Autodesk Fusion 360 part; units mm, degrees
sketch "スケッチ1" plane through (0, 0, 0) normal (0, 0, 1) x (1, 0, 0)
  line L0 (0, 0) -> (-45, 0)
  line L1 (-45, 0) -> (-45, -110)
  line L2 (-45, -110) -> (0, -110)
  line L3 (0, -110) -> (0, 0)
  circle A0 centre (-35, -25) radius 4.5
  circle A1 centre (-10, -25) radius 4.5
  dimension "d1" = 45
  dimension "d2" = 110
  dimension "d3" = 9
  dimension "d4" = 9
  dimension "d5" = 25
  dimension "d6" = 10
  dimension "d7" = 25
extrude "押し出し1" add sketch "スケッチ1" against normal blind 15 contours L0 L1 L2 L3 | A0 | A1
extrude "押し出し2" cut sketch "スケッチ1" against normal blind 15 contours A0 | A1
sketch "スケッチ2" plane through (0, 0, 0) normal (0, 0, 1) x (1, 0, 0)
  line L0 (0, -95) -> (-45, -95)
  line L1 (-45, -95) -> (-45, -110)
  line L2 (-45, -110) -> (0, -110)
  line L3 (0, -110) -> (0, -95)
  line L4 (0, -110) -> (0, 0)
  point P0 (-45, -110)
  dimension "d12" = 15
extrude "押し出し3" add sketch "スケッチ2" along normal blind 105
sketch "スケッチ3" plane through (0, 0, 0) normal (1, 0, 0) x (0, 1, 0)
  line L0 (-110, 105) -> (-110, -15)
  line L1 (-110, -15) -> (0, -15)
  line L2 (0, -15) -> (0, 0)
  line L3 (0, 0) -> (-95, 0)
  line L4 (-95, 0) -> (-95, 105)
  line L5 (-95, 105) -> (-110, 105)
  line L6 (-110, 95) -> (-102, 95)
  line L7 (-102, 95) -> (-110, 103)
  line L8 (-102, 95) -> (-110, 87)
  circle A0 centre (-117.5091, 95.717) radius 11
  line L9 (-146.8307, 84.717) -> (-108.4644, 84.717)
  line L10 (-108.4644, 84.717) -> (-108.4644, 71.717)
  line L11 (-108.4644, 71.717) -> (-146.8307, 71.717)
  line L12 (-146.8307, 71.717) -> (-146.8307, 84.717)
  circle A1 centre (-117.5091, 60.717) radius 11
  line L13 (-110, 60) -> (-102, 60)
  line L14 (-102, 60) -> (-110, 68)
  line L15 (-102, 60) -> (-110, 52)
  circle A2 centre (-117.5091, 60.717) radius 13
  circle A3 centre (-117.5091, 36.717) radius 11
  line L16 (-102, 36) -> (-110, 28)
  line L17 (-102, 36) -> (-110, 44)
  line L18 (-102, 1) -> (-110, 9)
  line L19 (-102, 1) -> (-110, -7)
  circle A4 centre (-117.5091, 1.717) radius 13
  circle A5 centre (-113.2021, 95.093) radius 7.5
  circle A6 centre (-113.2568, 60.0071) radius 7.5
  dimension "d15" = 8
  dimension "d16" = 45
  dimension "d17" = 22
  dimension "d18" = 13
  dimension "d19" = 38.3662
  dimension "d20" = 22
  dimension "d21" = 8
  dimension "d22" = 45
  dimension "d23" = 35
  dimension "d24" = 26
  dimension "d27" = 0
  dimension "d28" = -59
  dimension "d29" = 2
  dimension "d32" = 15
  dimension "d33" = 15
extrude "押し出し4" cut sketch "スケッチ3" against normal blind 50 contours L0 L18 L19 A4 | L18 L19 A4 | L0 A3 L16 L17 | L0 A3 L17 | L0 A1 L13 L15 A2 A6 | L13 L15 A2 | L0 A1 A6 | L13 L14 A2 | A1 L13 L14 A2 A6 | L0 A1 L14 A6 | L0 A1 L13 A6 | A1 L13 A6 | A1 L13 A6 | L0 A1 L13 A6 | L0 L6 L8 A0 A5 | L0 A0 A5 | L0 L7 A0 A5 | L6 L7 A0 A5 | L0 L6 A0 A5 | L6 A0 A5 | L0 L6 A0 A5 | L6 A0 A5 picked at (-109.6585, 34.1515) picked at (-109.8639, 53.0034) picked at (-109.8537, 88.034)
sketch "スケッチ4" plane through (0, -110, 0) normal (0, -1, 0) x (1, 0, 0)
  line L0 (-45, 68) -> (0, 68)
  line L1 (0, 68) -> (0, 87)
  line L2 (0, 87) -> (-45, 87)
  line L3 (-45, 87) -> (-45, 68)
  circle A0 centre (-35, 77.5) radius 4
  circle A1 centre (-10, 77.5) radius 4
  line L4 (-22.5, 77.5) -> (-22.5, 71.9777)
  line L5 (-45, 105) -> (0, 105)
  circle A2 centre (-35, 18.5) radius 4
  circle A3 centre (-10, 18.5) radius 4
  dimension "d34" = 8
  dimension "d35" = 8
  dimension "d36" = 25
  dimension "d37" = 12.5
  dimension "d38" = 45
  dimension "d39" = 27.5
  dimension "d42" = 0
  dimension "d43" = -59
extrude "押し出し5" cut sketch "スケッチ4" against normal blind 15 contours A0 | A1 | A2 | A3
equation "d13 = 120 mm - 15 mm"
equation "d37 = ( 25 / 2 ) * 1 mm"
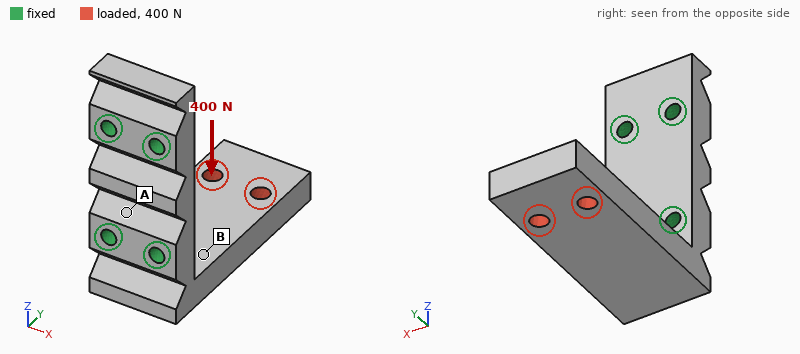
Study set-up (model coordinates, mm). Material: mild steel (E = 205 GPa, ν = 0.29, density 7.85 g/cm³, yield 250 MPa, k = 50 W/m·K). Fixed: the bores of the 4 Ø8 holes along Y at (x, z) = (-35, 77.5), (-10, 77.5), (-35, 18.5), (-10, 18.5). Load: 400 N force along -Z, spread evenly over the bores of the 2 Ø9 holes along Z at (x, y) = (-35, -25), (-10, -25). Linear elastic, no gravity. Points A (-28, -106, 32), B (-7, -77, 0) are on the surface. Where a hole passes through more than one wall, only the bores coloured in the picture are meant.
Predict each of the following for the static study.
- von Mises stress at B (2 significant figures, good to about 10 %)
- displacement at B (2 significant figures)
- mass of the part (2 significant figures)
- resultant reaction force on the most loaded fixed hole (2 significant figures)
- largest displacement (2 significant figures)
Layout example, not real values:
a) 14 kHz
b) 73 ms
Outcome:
a) 12 MPa
b) 0.020 mm
c) 1.0 kg
d) 190 N
e) 0.11 mm
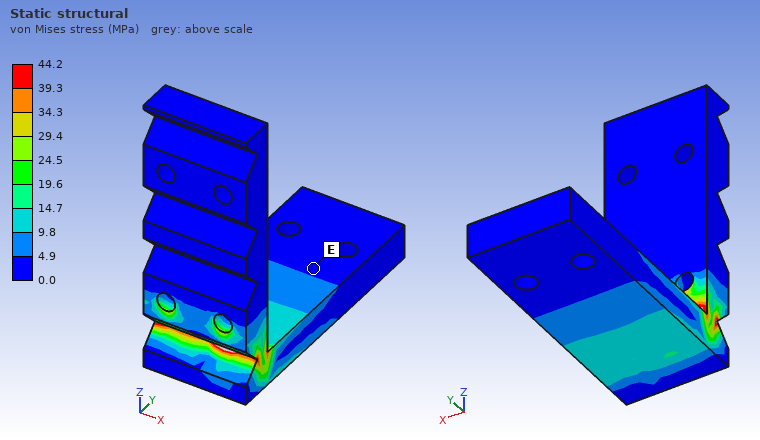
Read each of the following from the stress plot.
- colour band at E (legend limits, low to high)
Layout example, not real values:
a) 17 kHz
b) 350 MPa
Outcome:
a) 0.0 to 4.9 MPa
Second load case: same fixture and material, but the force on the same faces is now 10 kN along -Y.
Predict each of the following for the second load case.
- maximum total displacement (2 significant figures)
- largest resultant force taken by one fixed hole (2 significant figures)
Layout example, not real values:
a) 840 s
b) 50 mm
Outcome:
a) 0.31 mm
b) 5.1 kN
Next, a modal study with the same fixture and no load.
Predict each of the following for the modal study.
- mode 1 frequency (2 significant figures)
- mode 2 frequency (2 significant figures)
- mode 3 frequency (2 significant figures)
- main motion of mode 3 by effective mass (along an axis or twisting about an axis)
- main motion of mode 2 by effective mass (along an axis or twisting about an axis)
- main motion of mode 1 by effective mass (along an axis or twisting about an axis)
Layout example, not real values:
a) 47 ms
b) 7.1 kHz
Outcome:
a) 640 Hz
b) 1500 Hz
c) 4200 Hz
d) along Y
e) along X
f) along Z
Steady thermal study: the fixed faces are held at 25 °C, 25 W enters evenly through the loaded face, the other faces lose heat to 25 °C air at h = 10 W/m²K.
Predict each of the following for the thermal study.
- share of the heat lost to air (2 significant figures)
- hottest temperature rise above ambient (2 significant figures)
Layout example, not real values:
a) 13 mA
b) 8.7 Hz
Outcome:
a) 24 %
b) 65 K
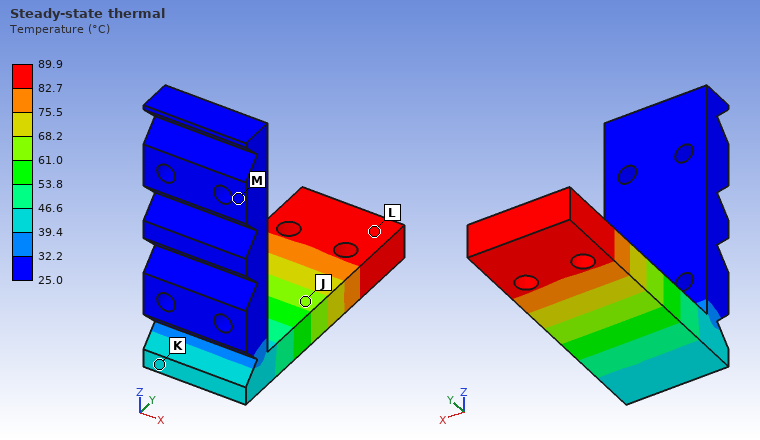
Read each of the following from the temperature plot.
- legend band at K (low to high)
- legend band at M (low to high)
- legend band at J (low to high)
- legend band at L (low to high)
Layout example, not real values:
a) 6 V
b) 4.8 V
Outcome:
a) 39.4 to 46.6 °C
b) 25.0 to 32.2 °C
c) 61.0 to 68.2 °C
d) 82.7 to 89.9 °C
